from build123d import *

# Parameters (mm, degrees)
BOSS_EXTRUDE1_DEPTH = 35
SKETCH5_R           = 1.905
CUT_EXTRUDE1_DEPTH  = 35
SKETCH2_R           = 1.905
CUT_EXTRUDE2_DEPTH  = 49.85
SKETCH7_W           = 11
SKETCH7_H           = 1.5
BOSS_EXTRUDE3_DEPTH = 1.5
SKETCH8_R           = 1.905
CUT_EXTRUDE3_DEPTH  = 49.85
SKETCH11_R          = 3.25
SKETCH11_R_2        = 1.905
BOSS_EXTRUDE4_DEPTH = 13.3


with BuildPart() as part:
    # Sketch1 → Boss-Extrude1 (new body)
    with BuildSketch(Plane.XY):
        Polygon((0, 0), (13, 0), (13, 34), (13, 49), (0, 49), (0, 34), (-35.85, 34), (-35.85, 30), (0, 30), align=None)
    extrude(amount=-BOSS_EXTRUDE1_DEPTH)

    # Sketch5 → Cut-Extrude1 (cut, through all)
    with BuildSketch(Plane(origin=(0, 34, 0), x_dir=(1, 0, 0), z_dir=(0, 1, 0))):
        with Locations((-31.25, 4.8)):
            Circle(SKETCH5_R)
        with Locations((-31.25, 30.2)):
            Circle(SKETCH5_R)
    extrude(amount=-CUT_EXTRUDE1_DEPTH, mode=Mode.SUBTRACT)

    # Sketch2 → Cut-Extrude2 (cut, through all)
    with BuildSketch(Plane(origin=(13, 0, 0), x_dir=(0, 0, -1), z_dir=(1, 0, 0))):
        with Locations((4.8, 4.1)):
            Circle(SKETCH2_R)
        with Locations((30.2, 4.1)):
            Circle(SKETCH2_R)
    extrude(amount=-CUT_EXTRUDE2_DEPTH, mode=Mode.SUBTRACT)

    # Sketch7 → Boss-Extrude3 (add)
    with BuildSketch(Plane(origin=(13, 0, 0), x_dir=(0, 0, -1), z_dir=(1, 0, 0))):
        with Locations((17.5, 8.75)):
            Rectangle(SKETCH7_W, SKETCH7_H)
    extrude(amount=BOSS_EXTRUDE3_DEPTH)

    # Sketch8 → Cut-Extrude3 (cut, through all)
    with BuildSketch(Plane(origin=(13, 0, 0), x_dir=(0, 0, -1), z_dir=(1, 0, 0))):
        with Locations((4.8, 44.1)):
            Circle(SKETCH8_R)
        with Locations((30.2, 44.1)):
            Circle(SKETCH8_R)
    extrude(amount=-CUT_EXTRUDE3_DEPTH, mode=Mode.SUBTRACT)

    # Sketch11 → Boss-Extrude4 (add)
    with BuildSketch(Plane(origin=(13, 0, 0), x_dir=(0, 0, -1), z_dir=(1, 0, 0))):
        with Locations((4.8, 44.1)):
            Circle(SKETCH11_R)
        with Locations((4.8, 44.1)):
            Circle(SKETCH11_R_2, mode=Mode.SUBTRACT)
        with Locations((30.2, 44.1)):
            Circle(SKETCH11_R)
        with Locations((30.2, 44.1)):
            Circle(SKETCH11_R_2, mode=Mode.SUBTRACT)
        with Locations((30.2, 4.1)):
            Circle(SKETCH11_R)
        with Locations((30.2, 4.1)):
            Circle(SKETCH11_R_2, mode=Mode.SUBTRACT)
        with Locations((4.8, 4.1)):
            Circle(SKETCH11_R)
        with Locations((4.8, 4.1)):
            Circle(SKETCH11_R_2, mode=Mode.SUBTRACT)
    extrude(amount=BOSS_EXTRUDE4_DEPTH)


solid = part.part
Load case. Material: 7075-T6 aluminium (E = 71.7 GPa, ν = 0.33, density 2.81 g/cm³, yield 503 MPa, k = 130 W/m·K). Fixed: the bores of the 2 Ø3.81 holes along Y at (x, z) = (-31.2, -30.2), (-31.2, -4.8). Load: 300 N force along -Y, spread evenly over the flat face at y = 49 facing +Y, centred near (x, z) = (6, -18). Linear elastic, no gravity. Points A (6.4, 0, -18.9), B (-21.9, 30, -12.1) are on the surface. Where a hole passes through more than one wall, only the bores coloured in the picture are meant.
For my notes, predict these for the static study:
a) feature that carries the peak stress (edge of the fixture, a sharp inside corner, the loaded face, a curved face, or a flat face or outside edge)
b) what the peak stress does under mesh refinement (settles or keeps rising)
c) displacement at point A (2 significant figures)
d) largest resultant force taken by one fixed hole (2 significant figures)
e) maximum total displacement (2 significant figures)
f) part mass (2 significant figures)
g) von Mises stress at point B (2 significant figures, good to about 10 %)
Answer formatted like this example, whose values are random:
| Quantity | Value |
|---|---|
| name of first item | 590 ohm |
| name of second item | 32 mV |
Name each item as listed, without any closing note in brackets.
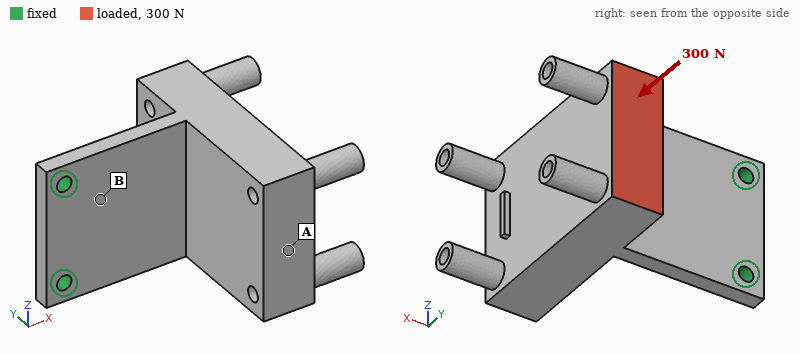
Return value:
| Quantity | Value |
|---|---|
| feature that carries the peak stress | edge of the fixture |
| what the peak stress does under mesh refinement | keeps rising |
| displacement at point A | 0.65 mm |
| largest resultant force taken by one fixed hole | 150 N |
| maximum total displacement | 0.88 mm |
| part mass | 78 g |
| von Mises stress at point B | 79 MPa |
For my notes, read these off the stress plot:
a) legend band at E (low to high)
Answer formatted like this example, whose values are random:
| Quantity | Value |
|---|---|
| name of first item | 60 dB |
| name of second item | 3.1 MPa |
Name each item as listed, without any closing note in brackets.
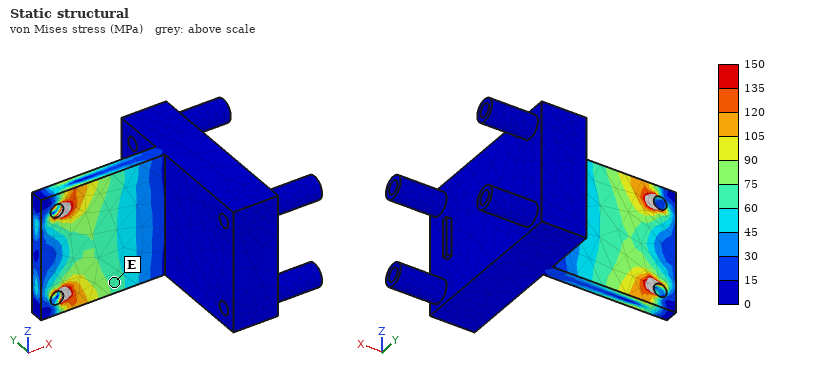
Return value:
| Quantity | Value |
|---|---|
| legend band at E | 60 to 75 MPa |
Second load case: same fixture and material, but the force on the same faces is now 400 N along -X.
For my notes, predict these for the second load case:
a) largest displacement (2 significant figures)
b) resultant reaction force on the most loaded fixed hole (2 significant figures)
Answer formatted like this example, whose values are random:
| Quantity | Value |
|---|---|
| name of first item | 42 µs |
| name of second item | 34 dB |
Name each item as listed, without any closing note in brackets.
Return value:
| Quantity | Value |
|---|---|
| largest displacement | 0.84 mm |
| resultant reaction force on the most loaded fixed hole | 200 N |
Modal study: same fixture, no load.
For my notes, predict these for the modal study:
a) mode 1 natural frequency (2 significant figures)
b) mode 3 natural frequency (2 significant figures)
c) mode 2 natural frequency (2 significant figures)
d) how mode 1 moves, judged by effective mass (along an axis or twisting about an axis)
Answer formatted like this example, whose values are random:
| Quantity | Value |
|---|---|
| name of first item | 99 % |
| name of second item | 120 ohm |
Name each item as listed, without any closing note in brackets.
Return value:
| Quantity | Value |
|---|---|
| mode 1 natural frequency | 430 Hz |
| mode 3 natural frequency | 2200 Hz |
| mode 2 natural frequency | 1100 Hz |
| how mode 1 moves, judged by effective mass | along Y |
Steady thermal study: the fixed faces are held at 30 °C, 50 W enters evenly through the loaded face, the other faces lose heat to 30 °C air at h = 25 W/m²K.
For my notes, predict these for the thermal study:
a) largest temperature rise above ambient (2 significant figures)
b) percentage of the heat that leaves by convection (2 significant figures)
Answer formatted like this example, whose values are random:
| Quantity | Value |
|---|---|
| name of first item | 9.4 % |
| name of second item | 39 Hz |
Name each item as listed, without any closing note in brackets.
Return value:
| Quantity | Value |
|---|---|
| largest temperature rise above ambient | 84 K |
| percentage of the heat that leaves by convection | 30 % |
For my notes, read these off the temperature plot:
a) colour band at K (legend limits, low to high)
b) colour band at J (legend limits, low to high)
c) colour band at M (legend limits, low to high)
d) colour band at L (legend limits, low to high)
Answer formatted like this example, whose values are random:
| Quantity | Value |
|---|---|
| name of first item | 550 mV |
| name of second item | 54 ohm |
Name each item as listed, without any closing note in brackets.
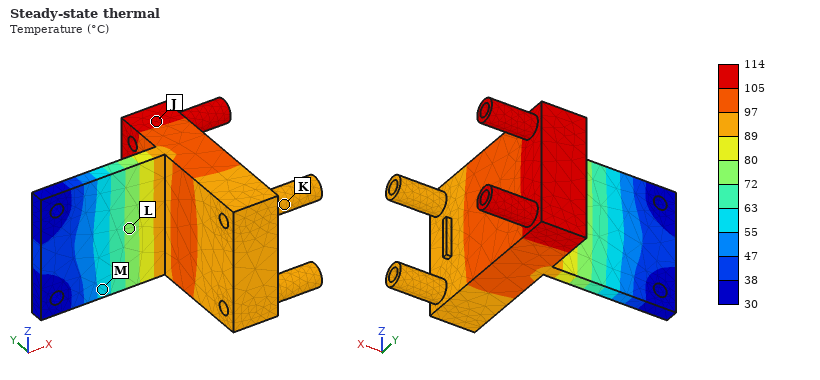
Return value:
| Quantity | Value |
|---|---|
| colour band at K | 89 to 97 °C |
| colour band at J | 105 to 114 °C |
| colour band at M | 55 to 63 °C |
| colour band at L | 72 to 80 °C |
